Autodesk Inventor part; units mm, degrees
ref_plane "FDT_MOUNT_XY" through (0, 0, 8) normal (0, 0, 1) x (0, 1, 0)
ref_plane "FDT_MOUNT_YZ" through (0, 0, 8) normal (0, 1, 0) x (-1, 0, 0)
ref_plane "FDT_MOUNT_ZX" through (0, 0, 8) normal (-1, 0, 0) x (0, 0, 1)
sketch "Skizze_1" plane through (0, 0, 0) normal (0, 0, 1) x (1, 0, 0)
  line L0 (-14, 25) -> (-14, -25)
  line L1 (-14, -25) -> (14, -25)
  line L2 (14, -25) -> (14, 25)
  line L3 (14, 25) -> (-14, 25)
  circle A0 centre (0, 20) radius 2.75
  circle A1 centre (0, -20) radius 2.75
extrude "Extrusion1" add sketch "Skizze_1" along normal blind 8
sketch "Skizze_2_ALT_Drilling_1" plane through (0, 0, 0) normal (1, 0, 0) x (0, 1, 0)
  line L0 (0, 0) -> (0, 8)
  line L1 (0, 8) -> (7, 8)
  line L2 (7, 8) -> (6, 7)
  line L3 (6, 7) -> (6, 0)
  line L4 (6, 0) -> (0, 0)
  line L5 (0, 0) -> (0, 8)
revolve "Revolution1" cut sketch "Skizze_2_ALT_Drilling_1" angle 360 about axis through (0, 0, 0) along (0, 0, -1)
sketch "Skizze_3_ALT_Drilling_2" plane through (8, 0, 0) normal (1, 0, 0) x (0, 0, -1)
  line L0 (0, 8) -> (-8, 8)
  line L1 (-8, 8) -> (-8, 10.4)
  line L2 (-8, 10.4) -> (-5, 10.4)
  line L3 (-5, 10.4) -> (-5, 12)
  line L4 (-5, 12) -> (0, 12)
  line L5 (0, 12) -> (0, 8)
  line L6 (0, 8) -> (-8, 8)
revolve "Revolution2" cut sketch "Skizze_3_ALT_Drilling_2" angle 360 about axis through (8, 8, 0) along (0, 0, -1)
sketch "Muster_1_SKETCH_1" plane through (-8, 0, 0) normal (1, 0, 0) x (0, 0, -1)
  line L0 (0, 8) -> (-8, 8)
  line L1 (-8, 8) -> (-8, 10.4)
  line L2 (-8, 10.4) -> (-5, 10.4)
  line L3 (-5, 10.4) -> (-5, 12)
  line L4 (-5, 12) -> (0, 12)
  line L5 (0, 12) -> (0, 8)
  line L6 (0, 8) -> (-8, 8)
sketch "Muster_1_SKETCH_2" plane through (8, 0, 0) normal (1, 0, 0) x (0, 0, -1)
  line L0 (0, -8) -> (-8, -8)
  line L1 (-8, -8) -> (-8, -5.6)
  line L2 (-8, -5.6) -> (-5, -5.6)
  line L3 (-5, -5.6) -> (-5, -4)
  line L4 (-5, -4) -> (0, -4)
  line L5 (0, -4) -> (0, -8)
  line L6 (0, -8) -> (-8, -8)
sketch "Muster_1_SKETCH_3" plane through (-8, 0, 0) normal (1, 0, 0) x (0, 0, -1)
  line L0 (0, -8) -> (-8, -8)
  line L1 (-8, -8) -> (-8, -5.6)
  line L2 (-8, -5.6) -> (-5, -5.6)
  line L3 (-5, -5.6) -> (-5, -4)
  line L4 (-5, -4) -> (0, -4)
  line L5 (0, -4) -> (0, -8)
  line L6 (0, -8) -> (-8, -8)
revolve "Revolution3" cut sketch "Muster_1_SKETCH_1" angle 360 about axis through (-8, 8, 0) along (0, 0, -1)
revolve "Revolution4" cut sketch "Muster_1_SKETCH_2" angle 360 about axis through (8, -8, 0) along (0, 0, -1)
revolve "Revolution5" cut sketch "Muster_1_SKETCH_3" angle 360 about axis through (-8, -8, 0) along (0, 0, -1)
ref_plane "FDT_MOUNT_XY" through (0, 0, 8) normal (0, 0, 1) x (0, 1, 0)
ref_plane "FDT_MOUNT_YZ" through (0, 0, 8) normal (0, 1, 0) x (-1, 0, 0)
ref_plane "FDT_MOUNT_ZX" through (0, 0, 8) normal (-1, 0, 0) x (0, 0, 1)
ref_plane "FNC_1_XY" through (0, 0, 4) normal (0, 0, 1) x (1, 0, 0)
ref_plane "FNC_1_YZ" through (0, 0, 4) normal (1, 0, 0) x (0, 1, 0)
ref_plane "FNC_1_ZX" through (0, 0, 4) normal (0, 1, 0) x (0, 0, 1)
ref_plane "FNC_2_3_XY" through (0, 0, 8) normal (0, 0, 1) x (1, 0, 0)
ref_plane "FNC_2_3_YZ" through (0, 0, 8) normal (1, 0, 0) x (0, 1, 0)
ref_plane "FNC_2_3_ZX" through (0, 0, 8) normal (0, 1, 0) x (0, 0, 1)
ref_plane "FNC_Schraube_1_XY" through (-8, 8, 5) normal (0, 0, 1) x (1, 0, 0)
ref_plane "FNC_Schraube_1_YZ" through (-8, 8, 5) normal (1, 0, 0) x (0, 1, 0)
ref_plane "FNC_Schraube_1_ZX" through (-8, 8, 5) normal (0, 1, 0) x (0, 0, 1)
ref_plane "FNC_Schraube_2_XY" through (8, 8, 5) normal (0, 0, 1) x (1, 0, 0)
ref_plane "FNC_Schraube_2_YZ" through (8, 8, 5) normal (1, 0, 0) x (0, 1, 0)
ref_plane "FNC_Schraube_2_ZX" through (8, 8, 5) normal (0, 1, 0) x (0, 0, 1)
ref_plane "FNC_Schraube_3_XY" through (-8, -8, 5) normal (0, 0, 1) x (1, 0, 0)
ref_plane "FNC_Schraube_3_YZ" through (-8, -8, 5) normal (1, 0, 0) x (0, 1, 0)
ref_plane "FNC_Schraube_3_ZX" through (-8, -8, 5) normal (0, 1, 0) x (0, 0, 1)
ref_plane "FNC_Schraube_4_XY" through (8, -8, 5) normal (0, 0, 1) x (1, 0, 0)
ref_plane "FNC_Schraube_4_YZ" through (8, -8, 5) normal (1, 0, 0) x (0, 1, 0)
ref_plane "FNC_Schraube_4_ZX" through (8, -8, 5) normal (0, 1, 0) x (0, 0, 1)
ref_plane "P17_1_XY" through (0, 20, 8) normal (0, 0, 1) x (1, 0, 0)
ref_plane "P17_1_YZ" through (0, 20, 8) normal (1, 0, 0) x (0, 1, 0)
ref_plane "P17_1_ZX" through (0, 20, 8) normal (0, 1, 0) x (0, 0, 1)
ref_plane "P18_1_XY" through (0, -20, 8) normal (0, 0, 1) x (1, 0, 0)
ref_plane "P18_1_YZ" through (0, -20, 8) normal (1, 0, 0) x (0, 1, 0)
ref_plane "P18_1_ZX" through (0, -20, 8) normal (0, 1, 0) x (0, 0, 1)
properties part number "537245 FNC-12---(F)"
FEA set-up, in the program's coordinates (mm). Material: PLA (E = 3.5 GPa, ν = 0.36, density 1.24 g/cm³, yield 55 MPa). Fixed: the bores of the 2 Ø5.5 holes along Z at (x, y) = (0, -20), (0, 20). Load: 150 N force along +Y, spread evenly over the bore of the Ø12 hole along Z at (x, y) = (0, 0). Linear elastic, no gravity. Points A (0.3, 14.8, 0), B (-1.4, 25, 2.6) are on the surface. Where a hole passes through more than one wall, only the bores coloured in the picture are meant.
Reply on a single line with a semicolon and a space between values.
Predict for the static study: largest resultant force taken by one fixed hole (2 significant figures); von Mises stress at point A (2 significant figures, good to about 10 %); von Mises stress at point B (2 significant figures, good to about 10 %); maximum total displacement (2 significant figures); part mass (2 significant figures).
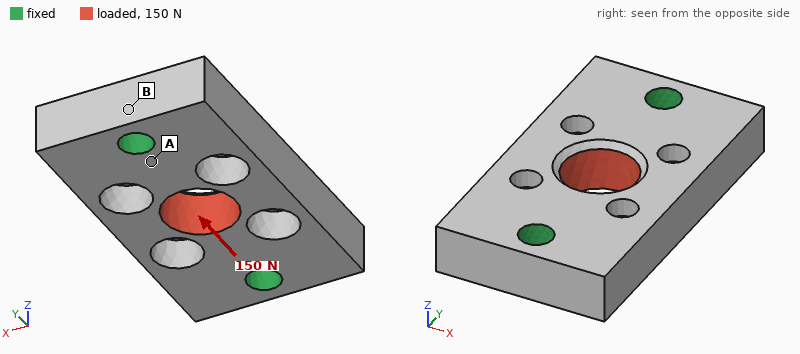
75 N; 1.1 MPa; 0.44 MPa; 7.4 µm; 11 g
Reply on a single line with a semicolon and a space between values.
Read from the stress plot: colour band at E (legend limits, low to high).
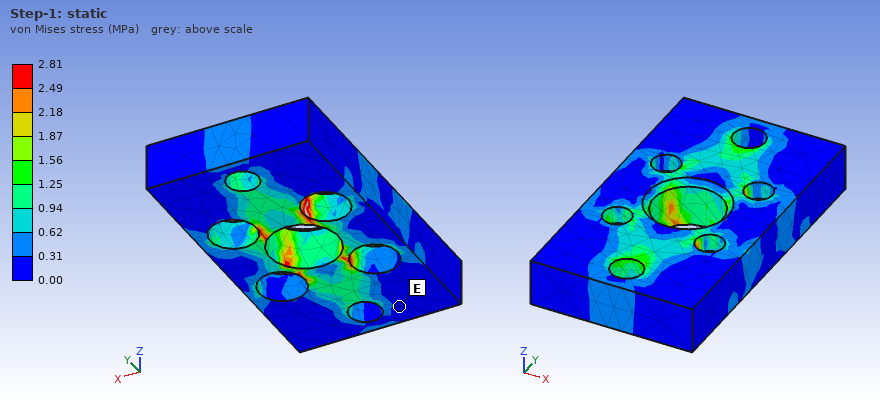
0.00 to 0.31 MPa
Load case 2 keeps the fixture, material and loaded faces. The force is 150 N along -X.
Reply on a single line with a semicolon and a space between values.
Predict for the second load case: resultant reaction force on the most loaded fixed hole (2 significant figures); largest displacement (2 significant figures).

75 N; 15 µm
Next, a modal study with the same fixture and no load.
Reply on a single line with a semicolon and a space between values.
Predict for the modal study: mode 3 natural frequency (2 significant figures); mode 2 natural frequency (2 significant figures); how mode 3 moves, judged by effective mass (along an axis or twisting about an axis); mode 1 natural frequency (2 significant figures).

9500 Hz; 6300 Hz; along X; 6100 Hz
